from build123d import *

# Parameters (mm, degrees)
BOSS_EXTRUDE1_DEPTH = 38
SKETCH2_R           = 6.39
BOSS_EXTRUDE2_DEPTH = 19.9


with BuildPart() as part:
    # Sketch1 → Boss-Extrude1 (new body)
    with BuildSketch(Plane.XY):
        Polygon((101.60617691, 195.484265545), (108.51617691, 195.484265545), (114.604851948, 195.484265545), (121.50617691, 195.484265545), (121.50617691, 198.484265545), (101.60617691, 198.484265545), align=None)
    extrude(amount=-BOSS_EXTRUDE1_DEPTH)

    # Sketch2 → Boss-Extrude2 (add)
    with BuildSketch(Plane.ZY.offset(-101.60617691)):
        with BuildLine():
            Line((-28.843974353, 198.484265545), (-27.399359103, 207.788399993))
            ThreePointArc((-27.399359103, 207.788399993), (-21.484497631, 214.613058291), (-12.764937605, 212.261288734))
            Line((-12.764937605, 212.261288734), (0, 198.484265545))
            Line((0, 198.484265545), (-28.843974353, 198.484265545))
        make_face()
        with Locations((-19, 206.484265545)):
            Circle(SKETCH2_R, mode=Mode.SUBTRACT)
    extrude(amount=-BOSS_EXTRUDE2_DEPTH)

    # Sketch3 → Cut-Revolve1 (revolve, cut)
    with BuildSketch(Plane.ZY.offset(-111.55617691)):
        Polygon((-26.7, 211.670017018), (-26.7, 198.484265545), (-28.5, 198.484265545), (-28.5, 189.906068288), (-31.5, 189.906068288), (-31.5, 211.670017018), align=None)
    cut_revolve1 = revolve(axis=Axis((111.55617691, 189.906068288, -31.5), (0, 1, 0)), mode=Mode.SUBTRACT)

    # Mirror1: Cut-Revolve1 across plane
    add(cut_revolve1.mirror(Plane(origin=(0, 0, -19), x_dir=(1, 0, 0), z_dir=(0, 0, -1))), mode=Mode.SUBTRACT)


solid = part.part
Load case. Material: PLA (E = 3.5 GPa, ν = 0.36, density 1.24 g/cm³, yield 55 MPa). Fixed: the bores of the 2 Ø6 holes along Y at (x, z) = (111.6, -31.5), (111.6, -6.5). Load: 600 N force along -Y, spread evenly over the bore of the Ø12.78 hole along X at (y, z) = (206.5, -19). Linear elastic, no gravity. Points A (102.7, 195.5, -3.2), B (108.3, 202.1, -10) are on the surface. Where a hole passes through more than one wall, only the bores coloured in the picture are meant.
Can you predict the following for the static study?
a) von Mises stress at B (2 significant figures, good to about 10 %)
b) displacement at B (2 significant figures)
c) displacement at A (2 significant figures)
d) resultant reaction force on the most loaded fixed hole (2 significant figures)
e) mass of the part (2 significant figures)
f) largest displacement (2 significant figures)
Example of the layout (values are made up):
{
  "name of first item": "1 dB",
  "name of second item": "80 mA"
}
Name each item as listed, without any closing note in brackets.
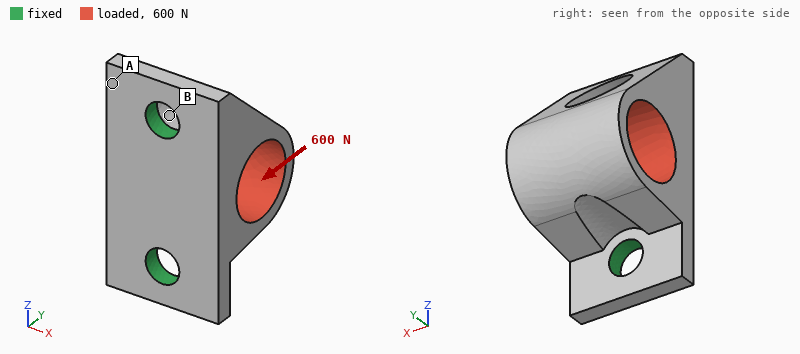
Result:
{
  "von Mises stress at B": "5.4 MPa",
  "displacement at B": "27 µm",
  "displacement at A": "13 µm",
  "resultant reaction force on the most loaded fixed hole": "330 N",
  "mass of the part": "6.5 g",
  "largest displacement": "62 µm"
}
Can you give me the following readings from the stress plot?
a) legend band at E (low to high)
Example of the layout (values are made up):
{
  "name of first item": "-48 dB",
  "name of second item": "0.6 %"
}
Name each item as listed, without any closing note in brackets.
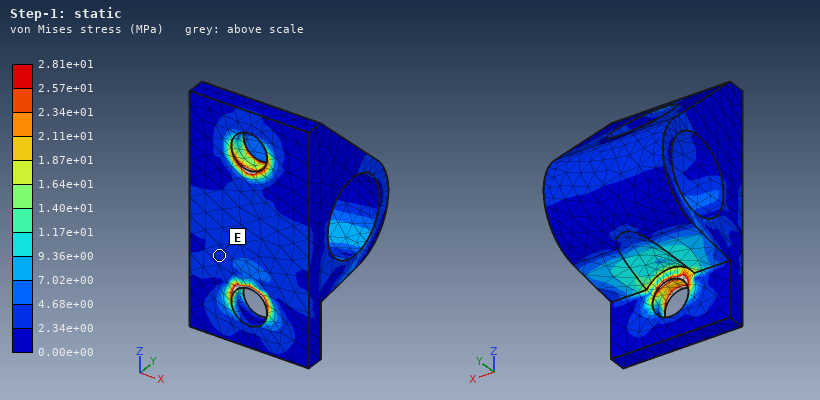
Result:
{
  "legend band at E": "2.34e+00 to 4.68e+00 MPa"
}
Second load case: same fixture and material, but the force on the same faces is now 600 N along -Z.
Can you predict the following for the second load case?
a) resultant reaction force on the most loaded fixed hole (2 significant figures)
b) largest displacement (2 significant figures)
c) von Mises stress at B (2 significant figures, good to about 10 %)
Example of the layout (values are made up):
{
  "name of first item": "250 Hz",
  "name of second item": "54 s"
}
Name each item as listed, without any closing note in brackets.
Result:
{
  "resultant reaction force on the most loaded fixed hole": "390 N",
  "largest displacement": "0.15 mm",
  "von Mises stress at B": "6.6 MPa"
}
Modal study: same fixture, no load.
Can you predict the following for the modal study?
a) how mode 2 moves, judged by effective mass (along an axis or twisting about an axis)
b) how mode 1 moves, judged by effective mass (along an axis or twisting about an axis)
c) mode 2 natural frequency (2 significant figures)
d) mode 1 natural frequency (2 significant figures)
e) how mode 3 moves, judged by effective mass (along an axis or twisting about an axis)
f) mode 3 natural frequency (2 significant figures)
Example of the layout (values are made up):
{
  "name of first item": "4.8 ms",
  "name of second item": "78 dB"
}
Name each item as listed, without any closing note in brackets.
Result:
{
  "how mode 2 moves, judged by effective mass": "along Z",
  "how mode 1 moves, judged by effective mass": "along X",
  "mode 2 natural frequency": "6700 Hz",
  "mode 1 natural frequency": "3600 Hz",
  "how mode 3 moves, judged by effective mass": "along Y",
  "mode 3 natural frequency": "8800 Hz"
}
